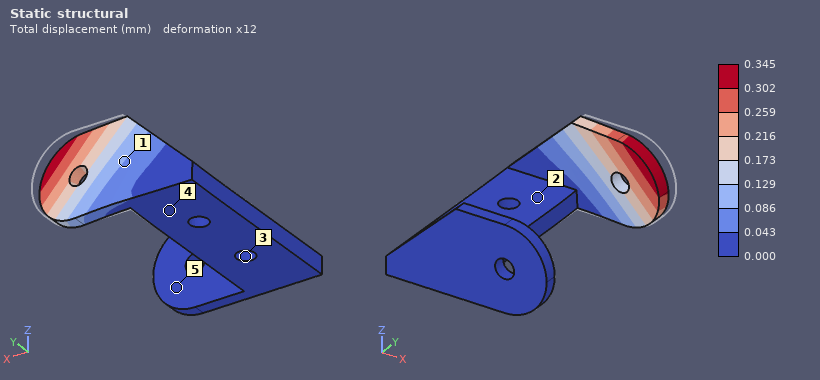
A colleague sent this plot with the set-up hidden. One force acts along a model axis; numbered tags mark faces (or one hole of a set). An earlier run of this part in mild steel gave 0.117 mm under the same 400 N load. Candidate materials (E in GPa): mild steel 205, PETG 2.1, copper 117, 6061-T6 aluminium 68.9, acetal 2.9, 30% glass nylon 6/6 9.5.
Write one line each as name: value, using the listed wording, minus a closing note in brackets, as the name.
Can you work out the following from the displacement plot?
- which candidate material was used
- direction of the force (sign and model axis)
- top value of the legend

which candidate material was used: 6061-T6 aluminium
direction of the force: -Y
top value of the legend: 0.345 mm
